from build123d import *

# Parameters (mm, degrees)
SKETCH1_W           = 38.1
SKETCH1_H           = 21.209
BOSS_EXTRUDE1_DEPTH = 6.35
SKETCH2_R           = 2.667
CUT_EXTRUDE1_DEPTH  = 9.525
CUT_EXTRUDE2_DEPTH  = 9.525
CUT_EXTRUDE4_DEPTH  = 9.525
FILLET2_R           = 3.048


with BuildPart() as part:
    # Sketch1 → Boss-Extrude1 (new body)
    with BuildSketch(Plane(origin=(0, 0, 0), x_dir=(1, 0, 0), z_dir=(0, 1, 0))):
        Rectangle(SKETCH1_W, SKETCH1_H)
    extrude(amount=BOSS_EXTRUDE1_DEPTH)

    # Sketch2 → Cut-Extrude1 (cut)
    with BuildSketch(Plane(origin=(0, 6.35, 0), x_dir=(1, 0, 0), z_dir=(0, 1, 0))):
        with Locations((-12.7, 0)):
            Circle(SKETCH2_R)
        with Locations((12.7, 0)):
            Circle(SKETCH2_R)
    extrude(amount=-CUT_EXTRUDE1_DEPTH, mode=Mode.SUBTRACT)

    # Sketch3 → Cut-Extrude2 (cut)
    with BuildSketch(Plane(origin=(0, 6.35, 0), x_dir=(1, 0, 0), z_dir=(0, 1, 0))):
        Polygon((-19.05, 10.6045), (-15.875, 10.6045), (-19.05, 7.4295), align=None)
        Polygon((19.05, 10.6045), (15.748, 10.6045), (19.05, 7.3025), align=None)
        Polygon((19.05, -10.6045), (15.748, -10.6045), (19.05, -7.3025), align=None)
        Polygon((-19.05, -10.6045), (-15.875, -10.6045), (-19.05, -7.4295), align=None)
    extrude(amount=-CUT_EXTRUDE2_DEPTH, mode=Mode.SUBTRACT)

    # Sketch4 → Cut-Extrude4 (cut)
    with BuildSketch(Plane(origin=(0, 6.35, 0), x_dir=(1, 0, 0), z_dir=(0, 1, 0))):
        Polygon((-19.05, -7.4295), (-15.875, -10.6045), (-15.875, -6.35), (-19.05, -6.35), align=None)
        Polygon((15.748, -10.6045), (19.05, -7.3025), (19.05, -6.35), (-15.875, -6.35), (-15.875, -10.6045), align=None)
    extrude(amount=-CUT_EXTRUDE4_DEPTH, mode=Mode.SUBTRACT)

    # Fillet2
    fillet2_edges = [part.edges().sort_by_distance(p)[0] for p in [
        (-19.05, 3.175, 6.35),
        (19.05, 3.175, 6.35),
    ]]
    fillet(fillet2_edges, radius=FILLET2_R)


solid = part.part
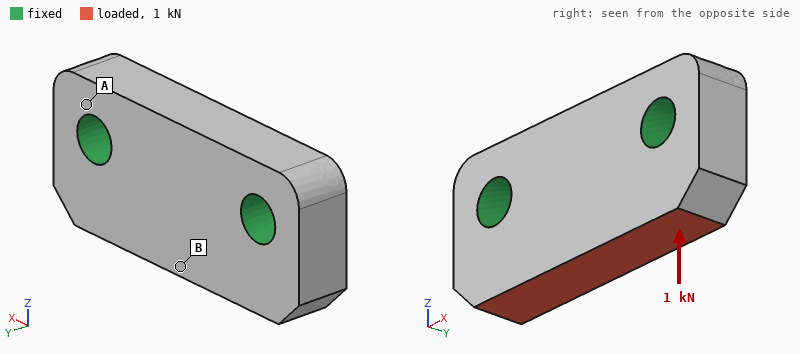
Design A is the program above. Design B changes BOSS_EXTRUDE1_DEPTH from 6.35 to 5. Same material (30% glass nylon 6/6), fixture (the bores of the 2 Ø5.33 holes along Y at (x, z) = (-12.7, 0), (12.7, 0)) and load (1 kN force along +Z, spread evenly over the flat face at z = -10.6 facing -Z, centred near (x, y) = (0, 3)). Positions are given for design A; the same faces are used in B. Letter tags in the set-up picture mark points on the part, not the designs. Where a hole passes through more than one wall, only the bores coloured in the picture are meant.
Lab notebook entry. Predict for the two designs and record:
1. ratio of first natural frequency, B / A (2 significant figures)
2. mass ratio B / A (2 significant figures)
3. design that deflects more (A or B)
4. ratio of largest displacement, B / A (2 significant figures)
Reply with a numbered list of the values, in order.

1. 0.87
2. 0.79
3. B
4. 1.3
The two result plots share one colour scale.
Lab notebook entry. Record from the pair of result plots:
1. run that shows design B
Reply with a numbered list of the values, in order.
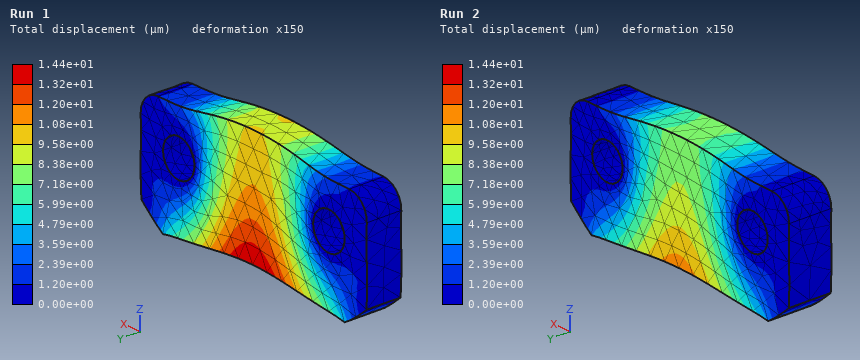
1. Run 1
